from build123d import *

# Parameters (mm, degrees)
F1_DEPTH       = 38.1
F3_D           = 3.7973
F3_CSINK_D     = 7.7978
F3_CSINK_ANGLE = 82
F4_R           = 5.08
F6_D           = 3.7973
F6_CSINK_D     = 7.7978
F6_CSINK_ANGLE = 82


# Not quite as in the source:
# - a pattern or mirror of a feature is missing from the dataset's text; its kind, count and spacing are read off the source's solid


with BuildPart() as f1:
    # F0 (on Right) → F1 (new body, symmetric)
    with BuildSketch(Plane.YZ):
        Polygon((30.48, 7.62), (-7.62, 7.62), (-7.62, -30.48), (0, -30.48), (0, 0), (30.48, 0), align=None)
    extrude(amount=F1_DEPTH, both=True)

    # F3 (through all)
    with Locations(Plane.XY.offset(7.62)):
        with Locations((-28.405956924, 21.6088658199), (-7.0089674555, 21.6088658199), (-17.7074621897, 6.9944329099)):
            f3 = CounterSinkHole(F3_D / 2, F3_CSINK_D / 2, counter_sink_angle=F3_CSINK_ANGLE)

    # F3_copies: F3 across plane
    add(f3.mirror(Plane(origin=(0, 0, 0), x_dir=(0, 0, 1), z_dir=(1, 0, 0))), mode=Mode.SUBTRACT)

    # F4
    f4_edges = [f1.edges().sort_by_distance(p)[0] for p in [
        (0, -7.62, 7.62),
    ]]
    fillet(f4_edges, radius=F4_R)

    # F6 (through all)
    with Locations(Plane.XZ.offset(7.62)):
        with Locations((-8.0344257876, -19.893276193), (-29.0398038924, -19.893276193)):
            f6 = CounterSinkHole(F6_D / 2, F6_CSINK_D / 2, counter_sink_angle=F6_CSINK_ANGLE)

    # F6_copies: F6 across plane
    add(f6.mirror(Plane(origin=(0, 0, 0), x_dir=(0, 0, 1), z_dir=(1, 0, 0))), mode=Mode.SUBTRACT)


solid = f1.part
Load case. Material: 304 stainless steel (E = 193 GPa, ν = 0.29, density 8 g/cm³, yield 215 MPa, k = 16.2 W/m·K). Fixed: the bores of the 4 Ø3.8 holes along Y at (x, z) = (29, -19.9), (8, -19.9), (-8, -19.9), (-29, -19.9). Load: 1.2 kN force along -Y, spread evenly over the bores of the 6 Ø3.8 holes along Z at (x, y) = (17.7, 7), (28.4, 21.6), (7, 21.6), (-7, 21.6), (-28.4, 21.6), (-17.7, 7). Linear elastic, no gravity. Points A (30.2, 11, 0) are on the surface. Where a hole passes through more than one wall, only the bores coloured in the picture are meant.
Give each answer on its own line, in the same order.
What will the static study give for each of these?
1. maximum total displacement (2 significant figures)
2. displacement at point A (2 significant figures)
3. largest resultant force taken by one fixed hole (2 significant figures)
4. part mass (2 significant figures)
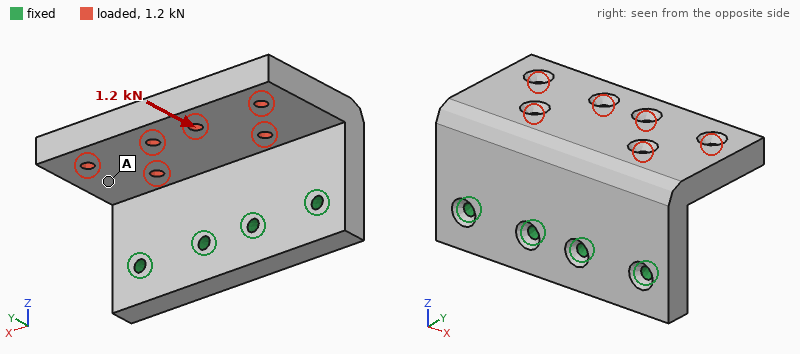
31 µm
16 µm
320 N
310 g
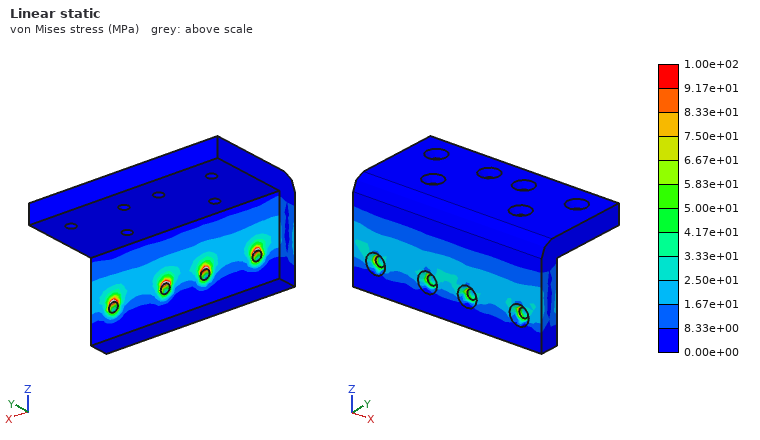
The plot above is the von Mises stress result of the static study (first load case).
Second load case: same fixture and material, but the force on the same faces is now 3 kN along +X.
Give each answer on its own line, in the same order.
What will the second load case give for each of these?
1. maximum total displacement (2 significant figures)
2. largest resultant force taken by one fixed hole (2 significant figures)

40 µm
1.6 kN
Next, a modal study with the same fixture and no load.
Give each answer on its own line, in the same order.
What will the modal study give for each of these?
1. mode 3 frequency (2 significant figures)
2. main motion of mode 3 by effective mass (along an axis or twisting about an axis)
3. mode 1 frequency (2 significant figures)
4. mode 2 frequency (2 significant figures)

6000 Hz
along Y
2200 Hz
3700 Hz
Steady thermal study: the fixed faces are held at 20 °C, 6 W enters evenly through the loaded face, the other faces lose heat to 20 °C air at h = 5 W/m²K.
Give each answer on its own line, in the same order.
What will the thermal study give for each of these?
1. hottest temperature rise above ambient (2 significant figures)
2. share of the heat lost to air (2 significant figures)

27 K
14 %
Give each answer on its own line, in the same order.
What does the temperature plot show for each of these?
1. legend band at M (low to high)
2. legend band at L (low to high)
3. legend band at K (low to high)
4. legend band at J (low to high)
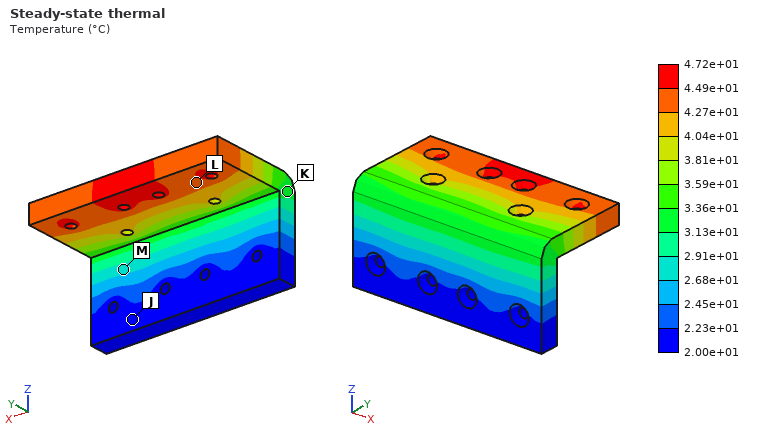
2.68e+01 to 2.91e+01 °C
4.27e+01 to 4.49e+01 °C
3.13e+01 to 3.36e+01 °C
2.00e+01 to 2.23e+01 °C
